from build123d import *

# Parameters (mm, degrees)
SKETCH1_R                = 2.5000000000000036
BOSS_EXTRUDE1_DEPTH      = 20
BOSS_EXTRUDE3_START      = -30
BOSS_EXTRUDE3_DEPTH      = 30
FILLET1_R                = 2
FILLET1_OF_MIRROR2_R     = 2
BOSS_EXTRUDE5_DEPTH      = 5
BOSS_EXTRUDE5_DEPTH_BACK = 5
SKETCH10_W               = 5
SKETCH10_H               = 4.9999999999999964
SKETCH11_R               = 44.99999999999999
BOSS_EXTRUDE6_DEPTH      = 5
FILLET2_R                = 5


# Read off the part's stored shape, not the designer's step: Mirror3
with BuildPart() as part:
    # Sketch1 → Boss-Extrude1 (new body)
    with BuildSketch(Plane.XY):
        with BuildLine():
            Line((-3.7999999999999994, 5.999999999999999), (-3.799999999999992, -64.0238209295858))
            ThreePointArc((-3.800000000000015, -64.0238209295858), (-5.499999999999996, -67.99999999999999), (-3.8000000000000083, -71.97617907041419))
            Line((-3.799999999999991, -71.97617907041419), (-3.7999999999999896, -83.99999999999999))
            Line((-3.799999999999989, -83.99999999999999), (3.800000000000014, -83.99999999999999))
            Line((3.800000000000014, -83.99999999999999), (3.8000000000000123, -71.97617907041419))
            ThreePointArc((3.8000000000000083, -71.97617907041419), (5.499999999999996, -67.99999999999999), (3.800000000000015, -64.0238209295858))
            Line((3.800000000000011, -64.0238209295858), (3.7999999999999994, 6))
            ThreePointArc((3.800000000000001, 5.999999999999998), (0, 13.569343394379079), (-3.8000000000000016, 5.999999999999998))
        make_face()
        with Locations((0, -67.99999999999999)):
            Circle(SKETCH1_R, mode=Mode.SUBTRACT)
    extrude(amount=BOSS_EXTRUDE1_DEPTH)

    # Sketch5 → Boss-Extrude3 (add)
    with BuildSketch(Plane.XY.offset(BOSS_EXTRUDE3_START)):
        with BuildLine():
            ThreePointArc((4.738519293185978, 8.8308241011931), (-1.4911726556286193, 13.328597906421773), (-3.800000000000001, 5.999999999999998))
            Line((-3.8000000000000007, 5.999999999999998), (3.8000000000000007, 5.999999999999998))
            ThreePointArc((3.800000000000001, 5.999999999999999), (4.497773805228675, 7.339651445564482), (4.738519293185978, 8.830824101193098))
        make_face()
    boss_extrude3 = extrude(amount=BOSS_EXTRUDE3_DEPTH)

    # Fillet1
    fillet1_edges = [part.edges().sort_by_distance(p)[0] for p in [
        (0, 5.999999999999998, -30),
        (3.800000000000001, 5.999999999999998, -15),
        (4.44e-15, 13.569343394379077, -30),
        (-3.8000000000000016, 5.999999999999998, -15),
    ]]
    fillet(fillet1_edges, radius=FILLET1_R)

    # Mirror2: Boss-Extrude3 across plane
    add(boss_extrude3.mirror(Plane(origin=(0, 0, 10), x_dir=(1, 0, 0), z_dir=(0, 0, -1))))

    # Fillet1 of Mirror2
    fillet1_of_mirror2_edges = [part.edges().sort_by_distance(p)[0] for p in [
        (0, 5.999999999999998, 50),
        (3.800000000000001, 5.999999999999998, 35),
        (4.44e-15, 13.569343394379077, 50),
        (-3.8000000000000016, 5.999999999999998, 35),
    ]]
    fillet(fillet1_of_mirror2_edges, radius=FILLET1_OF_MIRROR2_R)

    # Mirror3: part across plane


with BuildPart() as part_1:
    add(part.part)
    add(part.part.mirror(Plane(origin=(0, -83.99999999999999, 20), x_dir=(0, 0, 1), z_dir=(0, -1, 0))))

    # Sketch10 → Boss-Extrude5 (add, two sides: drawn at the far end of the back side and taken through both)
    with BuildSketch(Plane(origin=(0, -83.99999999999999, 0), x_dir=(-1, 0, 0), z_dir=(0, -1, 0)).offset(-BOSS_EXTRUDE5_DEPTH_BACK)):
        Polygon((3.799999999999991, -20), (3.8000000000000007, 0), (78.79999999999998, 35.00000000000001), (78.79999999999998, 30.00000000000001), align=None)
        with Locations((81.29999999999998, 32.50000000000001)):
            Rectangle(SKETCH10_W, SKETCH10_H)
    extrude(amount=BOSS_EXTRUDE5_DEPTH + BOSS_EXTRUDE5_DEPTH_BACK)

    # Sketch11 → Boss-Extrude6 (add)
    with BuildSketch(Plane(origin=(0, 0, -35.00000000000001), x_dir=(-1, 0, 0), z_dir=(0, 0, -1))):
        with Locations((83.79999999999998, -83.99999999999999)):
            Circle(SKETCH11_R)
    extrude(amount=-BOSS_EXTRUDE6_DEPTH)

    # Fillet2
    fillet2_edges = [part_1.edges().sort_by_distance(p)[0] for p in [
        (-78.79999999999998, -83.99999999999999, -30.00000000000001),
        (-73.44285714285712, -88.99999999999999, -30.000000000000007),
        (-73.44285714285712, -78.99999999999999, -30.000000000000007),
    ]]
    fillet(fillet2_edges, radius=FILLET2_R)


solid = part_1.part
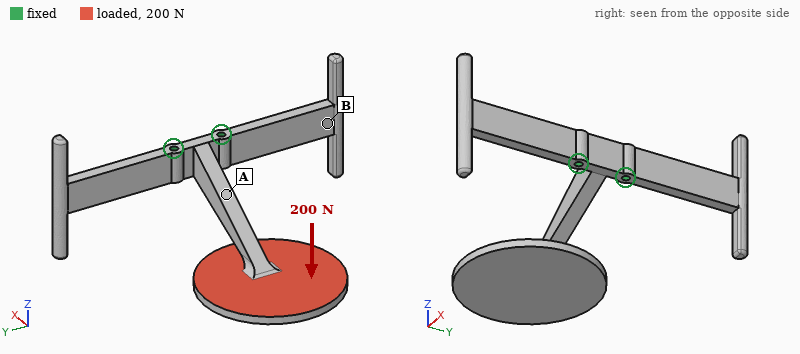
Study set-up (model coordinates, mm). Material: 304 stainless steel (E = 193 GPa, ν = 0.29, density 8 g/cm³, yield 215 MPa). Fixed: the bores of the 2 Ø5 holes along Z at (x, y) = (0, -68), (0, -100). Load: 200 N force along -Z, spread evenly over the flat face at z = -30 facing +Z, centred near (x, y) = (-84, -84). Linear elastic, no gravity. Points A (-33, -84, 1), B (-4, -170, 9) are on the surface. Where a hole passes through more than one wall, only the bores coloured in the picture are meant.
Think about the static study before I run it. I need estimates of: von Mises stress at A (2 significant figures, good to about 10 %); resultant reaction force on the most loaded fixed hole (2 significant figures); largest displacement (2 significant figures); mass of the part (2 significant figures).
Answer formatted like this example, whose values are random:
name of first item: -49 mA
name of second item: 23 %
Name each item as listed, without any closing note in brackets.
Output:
von Mises stress at A: 40 MPa
resultant reaction force on the most loaded fixed hole: 110 N
largest displacement: 0.35 mm
mass of the part: 620 g
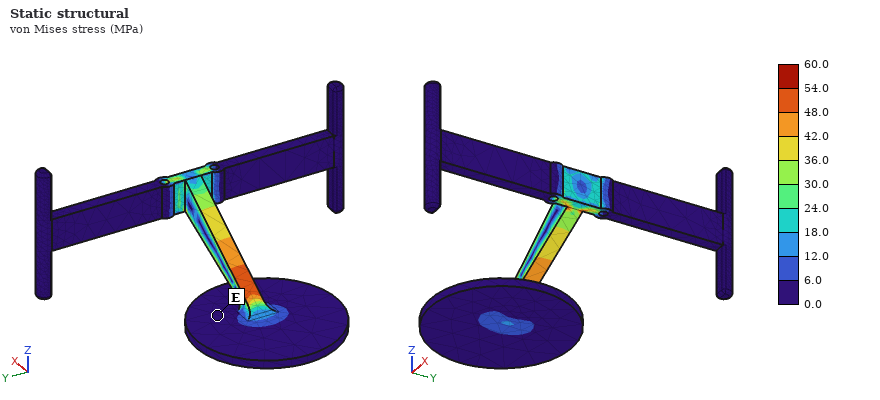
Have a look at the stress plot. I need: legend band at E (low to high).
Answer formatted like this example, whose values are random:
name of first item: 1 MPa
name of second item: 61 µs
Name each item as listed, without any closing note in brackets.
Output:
legend band at E: 0.0 to 6.0 MPa
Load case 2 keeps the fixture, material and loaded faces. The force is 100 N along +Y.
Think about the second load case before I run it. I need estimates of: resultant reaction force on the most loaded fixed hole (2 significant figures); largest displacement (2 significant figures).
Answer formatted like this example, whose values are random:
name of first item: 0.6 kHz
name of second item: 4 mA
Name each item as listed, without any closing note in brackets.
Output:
resultant reaction force on the most loaded fixed hole: 410 N
largest displacement: 0.22 mm
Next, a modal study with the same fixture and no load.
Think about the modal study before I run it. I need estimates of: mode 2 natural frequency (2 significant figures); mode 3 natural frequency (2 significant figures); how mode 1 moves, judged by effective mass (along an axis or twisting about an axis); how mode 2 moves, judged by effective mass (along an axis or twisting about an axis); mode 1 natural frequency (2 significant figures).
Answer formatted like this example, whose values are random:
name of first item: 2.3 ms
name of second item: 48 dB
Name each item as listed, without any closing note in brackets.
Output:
mode 2 natural frequency: 280 Hz
mode 3 natural frequency: 470 Hz
how mode 1 moves, judged by effective mass: along Y
how mode 2 moves, judged by effective mass: along Z
mode 1 natural frequency: 240 Hz
